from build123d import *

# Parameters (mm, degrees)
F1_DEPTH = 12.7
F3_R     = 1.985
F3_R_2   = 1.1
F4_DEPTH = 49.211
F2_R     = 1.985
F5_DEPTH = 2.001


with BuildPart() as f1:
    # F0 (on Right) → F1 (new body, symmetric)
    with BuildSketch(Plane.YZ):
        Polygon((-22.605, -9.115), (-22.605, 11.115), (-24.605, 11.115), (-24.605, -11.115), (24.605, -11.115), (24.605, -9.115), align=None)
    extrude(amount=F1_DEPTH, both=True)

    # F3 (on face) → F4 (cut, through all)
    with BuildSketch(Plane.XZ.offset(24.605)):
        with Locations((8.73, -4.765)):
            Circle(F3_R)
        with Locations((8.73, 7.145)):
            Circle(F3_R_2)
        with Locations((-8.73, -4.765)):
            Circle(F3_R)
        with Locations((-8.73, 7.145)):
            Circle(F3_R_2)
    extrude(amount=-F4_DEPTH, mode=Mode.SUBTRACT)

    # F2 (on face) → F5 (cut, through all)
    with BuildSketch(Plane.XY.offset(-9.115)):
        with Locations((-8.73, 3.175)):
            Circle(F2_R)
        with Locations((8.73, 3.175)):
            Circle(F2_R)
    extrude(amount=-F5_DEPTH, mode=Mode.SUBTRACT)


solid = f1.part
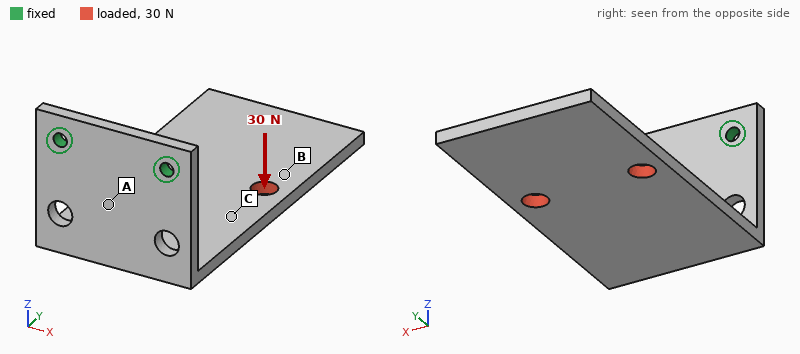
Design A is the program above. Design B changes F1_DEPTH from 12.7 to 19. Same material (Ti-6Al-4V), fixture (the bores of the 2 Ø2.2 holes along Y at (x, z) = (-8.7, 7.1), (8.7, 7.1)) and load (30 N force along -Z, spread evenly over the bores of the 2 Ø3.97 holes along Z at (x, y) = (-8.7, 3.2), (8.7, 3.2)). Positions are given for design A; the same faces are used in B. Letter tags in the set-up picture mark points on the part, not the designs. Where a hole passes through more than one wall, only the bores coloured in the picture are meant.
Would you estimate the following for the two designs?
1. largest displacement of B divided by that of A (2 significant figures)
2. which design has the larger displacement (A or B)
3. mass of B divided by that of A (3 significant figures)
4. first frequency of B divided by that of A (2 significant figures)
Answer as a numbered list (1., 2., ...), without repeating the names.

1. 0.67
2. A
3. 1.51
4. 1.0
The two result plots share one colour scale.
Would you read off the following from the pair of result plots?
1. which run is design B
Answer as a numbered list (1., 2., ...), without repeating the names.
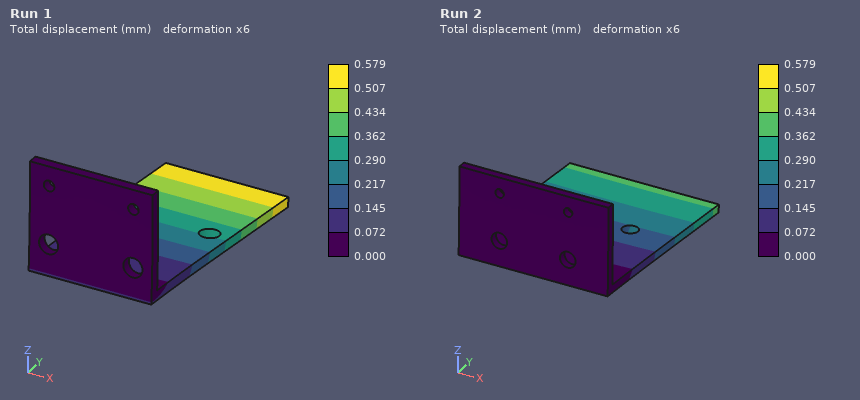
1. Run 2
